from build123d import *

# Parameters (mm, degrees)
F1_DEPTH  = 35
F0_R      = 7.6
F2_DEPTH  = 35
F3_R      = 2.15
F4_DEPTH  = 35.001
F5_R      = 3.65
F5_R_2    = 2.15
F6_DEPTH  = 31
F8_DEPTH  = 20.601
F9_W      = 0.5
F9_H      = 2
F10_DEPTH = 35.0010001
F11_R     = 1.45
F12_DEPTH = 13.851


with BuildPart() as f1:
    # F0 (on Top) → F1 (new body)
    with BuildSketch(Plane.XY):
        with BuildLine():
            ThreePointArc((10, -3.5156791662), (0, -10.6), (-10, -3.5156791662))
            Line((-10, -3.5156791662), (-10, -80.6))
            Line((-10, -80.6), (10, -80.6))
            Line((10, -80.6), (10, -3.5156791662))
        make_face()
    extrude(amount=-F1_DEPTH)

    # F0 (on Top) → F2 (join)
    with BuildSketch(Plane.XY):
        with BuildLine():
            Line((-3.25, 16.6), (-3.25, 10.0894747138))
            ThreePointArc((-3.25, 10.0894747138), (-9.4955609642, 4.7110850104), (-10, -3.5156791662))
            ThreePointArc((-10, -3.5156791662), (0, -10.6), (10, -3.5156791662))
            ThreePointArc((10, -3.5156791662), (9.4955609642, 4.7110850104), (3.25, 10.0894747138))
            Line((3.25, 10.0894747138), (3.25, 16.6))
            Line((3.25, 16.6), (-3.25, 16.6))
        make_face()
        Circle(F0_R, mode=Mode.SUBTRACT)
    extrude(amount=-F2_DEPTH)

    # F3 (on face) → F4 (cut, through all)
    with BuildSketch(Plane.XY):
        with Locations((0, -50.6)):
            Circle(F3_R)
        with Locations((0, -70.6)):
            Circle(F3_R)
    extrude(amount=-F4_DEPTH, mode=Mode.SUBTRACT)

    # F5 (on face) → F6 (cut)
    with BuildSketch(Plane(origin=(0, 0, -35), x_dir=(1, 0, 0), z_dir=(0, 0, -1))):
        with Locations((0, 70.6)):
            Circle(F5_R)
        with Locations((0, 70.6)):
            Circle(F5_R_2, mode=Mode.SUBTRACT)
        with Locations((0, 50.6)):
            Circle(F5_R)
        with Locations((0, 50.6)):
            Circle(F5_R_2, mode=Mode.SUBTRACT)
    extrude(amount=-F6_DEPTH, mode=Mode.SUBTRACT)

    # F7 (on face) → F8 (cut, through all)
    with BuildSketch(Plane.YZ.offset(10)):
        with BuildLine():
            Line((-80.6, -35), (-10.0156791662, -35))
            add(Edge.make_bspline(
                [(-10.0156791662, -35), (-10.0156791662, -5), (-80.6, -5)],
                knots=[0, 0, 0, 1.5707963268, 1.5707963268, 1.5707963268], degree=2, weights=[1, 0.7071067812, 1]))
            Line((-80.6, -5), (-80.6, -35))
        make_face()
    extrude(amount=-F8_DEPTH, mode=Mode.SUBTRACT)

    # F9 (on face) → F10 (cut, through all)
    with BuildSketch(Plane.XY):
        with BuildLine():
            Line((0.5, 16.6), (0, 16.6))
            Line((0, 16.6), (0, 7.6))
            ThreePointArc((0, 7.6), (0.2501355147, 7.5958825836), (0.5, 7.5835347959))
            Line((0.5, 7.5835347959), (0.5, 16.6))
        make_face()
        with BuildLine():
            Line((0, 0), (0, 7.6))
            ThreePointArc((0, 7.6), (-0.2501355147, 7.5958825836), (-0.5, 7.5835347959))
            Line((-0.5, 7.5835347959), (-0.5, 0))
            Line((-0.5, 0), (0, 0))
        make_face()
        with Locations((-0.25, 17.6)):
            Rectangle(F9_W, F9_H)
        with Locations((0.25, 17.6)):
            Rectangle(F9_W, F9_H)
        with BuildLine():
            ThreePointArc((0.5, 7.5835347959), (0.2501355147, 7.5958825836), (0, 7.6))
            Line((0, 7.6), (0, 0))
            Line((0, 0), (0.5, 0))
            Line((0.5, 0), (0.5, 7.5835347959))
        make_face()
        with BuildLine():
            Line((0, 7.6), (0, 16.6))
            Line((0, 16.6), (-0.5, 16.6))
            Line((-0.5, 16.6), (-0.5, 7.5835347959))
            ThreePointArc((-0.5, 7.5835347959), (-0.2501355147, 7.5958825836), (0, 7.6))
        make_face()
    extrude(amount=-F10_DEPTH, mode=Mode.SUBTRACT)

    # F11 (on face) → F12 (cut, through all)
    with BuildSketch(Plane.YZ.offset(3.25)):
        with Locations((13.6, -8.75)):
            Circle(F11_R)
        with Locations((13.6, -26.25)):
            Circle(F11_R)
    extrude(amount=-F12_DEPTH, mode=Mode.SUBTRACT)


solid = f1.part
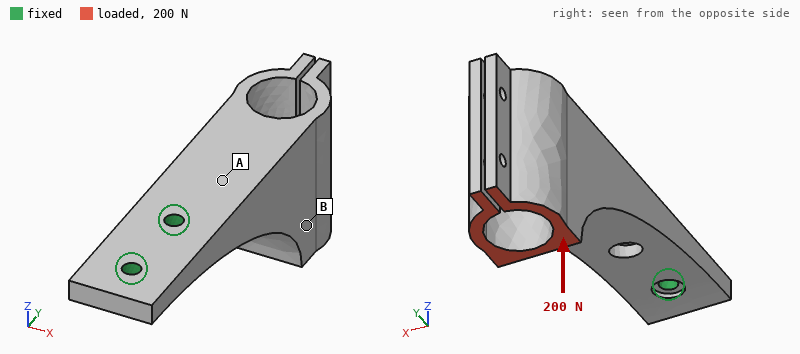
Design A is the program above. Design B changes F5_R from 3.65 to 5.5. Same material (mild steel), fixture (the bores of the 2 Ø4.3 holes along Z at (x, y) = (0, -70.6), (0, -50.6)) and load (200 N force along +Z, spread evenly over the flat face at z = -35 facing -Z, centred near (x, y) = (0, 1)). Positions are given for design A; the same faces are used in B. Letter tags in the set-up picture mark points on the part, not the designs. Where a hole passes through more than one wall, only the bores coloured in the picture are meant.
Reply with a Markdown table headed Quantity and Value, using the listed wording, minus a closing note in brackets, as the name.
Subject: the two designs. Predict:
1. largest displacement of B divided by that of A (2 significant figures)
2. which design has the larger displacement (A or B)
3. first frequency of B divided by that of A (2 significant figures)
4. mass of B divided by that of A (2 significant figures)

| Quantity | Value |
|---|---|
| largest displacement of B divided by that of A | 1.2 |
| which design has the larger displacement | B |
| first frequency of B divided by that of A | 0.92 |
| mass of B divided by that of A | 0.99 |
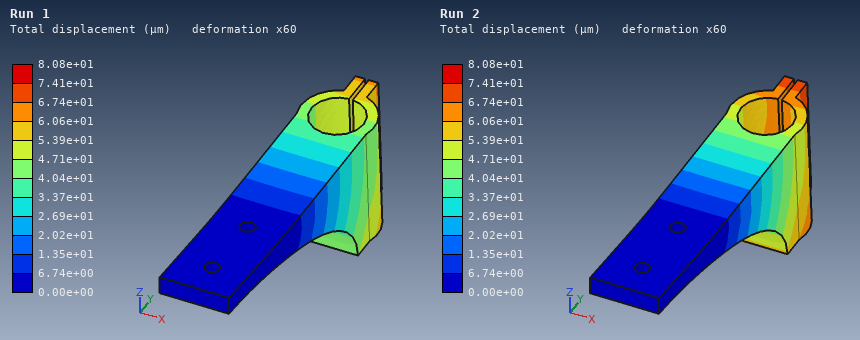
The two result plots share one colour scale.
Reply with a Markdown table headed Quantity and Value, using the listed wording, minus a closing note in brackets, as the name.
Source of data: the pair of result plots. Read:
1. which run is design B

| Quantity | Value |
|---|---|
| which run is design B | Run 2 |
